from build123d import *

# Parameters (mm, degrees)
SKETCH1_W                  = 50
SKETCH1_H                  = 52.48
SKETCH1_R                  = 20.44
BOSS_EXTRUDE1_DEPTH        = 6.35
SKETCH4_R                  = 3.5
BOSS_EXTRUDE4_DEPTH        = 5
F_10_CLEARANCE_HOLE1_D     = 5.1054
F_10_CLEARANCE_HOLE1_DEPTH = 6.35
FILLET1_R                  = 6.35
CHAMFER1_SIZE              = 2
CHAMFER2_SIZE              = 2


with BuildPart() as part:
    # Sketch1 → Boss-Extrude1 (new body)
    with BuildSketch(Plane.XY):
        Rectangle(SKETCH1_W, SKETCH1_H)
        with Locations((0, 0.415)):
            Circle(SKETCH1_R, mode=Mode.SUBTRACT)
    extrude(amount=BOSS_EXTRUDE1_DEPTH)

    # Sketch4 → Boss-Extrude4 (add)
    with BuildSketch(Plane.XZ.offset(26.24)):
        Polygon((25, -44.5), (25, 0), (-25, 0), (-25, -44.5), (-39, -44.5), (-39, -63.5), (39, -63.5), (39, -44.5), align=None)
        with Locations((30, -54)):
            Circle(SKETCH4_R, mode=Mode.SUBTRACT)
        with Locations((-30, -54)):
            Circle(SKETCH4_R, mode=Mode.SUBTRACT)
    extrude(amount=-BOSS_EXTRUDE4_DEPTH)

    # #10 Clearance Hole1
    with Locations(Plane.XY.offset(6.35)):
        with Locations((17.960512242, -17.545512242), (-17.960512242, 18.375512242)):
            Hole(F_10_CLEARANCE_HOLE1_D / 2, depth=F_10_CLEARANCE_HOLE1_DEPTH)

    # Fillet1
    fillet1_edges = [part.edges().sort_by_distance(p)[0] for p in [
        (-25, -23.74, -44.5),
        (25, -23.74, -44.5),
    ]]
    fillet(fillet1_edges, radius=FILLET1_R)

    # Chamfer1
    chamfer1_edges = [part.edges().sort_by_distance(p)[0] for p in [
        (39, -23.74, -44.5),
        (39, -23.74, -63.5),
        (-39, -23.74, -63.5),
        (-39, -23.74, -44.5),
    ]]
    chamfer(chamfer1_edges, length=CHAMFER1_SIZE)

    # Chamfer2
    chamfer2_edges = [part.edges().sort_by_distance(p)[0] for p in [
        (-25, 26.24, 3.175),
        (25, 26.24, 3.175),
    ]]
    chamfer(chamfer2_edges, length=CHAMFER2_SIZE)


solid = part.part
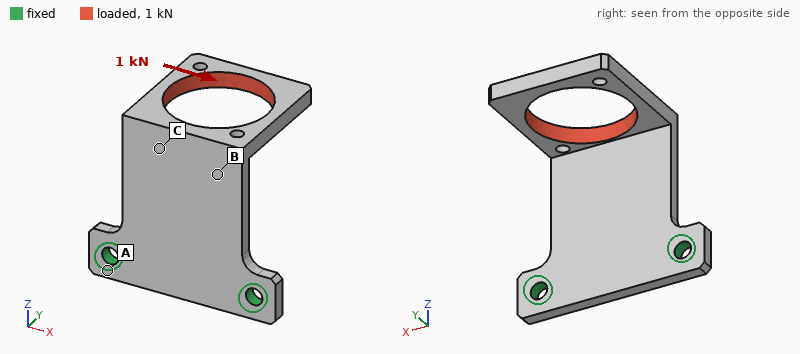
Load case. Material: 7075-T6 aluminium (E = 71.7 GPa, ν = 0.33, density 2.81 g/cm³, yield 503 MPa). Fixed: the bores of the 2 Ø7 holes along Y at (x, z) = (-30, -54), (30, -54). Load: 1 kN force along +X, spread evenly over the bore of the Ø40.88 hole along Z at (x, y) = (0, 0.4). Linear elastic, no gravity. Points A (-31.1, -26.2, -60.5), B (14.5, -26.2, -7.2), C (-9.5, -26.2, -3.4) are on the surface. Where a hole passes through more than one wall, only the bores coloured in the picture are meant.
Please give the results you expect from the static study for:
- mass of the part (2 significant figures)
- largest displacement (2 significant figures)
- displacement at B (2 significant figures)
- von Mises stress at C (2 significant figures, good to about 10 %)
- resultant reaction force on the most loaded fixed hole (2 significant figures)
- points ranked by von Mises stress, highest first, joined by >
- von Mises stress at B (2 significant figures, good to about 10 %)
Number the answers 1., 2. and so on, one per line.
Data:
1. 74 g
2. 1.0 mm
3. 0.20 mm
4. 63 MPa
5. 1.2 kN
6. B > C > A
7. 78 MPa
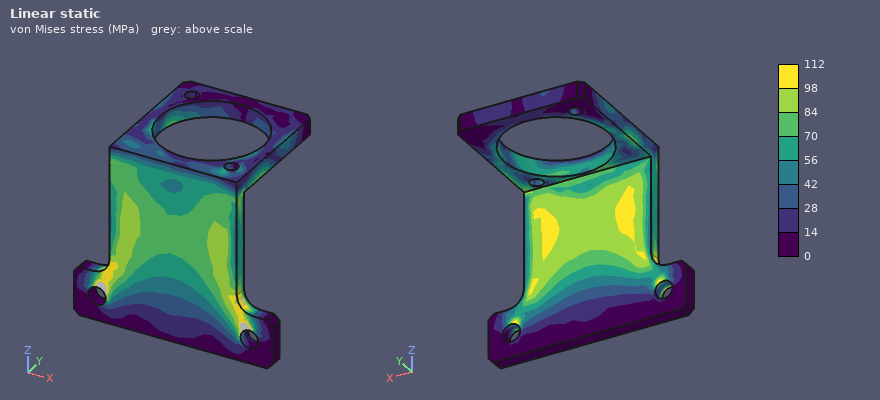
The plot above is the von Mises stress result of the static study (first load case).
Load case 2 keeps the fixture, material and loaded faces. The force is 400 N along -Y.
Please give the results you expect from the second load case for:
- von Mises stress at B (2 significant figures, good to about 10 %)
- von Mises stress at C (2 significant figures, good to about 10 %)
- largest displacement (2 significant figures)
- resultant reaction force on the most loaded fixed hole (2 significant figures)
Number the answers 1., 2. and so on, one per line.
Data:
1. 24 MPa
2. 16 MPa
3. 1.3 mm
4. 200 N
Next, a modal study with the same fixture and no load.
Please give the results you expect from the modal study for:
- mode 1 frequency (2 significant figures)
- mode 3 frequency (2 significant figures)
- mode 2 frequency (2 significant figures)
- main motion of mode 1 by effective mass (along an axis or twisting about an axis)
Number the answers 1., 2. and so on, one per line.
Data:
1. 530 Hz
2. 1300 Hz
3. 1100 Hz
4. along Y
